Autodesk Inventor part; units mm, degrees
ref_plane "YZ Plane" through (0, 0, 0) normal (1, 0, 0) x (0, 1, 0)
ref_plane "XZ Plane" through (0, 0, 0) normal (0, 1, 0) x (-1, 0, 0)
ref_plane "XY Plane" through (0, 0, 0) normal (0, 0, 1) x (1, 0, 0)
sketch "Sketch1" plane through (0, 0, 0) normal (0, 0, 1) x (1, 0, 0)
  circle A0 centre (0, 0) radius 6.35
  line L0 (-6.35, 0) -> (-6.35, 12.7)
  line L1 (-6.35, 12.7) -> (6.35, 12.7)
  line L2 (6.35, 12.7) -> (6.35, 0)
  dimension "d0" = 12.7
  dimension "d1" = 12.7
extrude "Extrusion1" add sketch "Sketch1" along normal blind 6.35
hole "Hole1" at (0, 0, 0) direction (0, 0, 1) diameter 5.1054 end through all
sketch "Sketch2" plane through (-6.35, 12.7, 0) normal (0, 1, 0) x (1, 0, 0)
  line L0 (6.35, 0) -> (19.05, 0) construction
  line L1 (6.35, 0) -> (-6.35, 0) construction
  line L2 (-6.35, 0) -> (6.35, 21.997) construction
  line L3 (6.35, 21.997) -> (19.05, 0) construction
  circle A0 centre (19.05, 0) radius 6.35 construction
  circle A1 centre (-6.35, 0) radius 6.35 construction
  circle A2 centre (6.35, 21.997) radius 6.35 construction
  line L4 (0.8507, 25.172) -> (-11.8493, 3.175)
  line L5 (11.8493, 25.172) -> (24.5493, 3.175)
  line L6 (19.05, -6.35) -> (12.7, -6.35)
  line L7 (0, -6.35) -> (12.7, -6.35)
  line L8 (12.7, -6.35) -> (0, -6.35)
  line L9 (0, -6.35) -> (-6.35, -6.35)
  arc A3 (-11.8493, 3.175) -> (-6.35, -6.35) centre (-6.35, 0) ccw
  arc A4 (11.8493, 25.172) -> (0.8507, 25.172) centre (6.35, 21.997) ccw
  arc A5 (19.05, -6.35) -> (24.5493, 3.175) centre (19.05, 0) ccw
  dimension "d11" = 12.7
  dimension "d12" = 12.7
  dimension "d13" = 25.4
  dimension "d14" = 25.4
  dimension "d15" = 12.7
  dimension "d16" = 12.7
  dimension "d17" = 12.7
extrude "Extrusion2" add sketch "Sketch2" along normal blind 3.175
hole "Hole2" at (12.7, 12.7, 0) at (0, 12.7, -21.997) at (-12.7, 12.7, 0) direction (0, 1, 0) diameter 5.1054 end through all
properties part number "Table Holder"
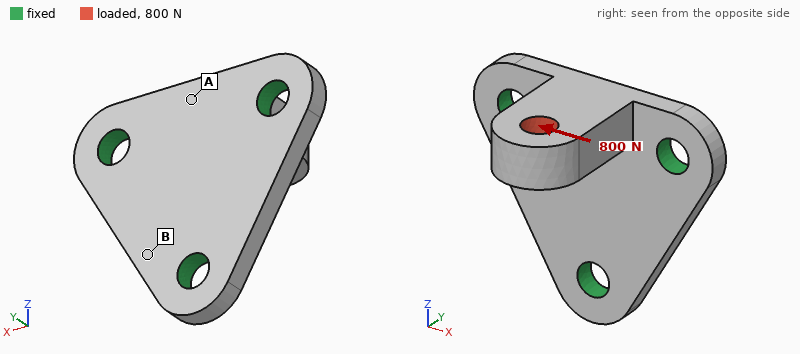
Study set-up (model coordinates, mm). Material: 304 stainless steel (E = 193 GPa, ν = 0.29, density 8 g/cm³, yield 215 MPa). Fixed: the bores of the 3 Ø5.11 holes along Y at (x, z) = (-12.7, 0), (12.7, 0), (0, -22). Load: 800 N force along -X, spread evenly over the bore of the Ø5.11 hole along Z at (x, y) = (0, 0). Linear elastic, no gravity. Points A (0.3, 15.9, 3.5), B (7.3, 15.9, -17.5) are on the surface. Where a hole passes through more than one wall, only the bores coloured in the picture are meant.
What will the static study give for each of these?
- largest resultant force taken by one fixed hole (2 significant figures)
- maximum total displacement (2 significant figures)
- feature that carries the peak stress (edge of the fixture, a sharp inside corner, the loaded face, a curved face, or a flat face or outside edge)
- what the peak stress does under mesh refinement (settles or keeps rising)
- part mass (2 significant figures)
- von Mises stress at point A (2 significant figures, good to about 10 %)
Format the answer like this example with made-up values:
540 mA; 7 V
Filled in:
770 N; 21 µm; edge of the fixture; keeps rising; 31 g; 21 MPa
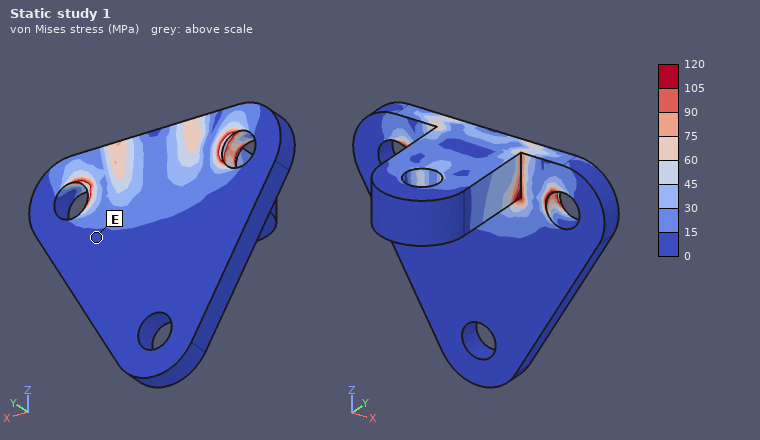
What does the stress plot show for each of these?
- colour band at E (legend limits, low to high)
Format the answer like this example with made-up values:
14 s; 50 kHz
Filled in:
0 to 15 MPa
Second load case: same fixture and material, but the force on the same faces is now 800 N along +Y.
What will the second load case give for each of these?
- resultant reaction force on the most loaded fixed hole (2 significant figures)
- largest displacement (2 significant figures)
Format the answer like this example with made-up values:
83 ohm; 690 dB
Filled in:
430 N; 13 µm
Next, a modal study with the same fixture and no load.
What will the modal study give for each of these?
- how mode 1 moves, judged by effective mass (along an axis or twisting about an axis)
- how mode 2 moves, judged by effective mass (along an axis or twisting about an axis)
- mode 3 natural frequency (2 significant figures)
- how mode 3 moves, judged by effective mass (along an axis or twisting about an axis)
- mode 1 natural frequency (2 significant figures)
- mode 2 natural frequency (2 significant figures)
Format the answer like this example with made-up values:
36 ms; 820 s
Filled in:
along Z; along X; 20 kHz; along Y; 7000 Hz; 14 kHz
